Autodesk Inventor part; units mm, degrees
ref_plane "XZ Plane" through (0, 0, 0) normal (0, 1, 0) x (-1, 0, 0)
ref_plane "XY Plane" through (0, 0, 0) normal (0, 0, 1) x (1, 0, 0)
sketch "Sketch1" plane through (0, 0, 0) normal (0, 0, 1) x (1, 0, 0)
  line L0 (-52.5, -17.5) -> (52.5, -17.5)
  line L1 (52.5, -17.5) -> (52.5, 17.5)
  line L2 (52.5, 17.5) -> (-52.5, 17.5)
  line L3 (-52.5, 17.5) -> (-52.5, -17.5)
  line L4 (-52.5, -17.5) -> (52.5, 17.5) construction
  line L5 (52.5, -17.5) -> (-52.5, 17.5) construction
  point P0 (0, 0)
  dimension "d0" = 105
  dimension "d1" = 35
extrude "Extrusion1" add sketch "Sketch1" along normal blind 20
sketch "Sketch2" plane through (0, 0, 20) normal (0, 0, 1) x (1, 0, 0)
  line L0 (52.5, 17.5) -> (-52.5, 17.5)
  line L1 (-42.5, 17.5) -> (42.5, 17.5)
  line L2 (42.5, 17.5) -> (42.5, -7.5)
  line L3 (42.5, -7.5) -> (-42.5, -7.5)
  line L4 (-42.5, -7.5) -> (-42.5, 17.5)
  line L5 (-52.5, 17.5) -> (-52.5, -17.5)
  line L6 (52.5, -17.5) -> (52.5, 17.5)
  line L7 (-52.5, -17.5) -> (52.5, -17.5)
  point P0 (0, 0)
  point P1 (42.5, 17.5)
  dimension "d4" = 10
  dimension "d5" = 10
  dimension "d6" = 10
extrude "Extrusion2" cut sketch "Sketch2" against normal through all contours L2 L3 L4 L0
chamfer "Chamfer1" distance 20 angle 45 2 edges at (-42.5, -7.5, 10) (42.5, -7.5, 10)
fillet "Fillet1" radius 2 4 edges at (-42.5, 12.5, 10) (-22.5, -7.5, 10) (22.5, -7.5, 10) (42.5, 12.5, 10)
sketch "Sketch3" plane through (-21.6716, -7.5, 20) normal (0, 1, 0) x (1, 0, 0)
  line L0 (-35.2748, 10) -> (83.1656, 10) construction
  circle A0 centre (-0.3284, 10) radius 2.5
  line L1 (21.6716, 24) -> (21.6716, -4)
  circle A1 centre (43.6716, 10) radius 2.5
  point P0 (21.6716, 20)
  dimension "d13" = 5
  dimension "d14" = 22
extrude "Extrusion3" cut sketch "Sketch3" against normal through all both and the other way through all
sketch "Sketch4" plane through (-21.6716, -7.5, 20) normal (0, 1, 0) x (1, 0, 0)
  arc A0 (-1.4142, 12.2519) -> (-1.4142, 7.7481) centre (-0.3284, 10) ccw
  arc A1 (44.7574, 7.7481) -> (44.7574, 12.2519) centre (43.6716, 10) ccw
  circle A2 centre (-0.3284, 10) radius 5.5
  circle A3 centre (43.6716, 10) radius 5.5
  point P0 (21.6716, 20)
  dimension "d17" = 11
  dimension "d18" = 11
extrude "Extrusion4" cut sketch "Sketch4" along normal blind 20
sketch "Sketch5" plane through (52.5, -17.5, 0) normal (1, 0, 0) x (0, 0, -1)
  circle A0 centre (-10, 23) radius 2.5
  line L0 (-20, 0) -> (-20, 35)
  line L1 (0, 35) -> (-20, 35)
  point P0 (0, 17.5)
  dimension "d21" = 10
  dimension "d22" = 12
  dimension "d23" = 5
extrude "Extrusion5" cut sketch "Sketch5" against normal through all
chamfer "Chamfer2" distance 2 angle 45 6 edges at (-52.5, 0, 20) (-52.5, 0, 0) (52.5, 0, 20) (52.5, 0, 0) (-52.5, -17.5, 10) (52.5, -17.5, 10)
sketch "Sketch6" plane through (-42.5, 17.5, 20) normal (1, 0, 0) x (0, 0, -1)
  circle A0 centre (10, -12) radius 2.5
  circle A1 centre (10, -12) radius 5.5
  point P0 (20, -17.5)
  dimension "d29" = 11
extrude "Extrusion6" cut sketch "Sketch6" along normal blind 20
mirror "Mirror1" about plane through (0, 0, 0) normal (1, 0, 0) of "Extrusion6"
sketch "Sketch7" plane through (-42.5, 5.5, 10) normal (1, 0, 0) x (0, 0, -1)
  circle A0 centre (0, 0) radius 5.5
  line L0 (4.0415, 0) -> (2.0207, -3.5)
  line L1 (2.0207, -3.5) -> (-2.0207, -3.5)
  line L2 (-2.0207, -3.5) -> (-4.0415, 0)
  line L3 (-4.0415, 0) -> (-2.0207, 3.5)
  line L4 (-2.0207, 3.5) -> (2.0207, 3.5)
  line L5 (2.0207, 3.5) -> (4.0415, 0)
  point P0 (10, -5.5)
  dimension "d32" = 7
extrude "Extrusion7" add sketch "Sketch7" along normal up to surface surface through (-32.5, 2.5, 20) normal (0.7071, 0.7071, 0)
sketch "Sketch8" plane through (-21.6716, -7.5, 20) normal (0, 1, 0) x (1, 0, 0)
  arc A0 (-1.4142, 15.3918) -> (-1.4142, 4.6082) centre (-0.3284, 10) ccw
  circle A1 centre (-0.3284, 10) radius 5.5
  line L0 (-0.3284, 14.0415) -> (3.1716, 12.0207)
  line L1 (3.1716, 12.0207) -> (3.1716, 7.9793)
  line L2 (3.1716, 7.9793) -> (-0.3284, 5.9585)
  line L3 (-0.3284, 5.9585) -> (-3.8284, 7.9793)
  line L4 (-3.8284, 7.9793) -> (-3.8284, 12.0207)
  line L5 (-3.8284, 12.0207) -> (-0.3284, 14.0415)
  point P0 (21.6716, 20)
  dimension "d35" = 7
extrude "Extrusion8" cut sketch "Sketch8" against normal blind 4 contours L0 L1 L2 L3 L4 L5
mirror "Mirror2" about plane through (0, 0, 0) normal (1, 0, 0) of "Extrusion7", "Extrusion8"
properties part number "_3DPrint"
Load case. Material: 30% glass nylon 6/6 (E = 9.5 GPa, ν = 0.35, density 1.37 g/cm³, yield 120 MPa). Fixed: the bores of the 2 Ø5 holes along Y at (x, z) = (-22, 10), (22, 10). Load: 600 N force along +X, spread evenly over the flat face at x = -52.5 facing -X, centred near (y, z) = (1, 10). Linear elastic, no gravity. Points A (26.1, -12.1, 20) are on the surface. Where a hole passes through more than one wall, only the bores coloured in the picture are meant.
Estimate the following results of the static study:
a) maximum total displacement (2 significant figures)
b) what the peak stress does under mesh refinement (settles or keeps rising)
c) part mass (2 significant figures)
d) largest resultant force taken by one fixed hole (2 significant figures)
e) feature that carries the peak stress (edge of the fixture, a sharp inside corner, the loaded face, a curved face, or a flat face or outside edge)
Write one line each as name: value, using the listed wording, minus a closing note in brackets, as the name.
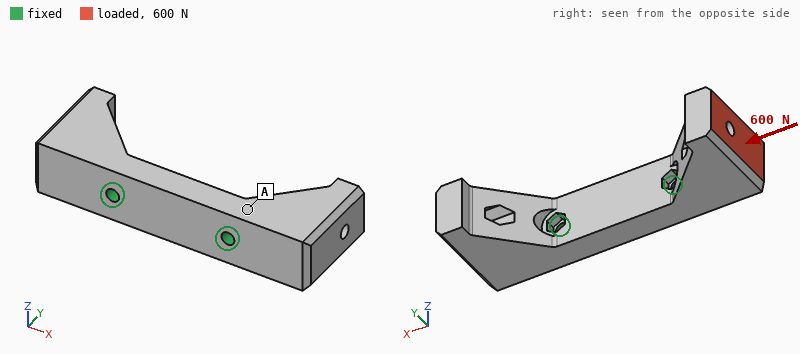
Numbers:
maximum total displacement: 0.30 mm
what the peak stress does under mesh refinement: keeps rising
part mass: 51 g
largest resultant force taken by one fixed hole: 320 N
feature that carries the peak stress: edge of the fixture
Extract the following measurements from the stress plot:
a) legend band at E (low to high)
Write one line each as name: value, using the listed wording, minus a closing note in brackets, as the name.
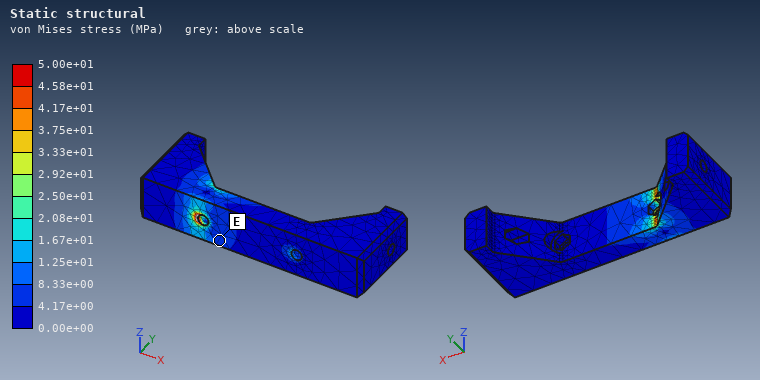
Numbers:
legend band at E: 4.17e+00 to 8.33e+00 MPa
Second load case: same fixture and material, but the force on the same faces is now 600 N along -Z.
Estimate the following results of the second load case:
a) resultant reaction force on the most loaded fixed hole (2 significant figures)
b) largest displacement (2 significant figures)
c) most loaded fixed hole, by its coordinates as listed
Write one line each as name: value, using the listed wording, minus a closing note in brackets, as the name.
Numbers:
resultant reaction force on the most loaded fixed hole: 890 N
largest displacement: 0.40 mm
most loaded fixed hole, by its coordinates as listed: (-22, 10)
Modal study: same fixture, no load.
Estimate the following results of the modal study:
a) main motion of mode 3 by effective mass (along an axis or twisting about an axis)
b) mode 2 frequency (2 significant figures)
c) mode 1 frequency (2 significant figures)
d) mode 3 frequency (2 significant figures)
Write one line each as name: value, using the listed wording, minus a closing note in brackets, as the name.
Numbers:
main motion of mode 3 by effective mass: along Z
mode 2 frequency: 1800 Hz
mode 1 frequency: 1800 Hz
mode 3 frequency: 2200 Hz
